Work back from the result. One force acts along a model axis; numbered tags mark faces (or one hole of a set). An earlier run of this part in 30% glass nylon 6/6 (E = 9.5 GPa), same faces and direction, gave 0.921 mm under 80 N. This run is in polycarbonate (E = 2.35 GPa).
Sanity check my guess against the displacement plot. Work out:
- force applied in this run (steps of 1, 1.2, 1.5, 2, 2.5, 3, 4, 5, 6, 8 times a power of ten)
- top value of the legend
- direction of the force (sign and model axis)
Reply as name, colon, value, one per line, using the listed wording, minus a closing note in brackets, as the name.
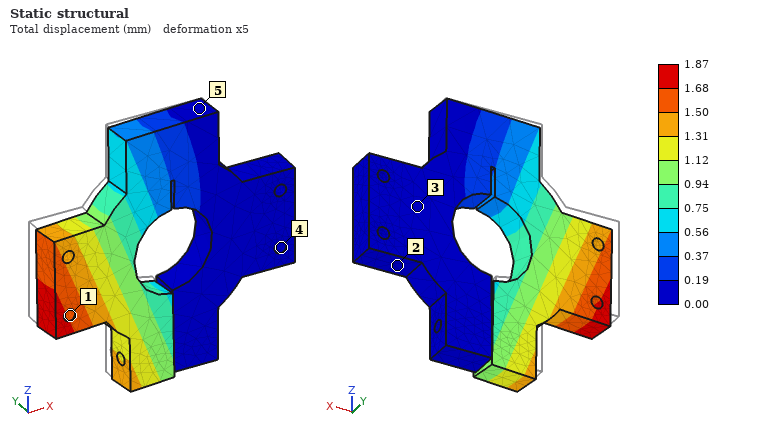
force applied in this run: 40 N
top value of the legend: 1.87 mm
direction of the force: -Y
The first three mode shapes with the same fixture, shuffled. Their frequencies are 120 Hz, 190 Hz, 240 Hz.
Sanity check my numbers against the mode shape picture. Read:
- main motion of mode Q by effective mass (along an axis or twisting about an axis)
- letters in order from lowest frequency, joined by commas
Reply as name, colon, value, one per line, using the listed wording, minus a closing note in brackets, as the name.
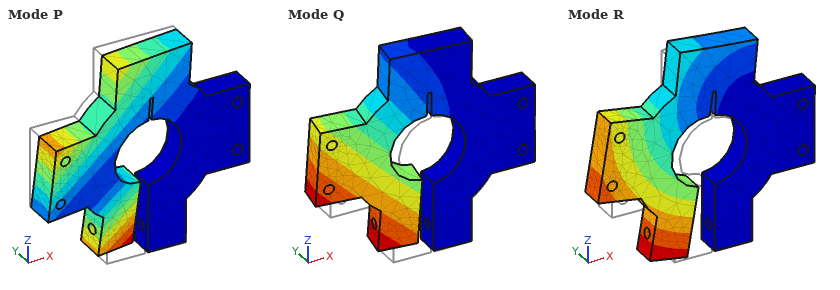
main motion of mode Q by effective mass: along Y
letters in order from lowest frequency, joined by commas: Q, R, P
